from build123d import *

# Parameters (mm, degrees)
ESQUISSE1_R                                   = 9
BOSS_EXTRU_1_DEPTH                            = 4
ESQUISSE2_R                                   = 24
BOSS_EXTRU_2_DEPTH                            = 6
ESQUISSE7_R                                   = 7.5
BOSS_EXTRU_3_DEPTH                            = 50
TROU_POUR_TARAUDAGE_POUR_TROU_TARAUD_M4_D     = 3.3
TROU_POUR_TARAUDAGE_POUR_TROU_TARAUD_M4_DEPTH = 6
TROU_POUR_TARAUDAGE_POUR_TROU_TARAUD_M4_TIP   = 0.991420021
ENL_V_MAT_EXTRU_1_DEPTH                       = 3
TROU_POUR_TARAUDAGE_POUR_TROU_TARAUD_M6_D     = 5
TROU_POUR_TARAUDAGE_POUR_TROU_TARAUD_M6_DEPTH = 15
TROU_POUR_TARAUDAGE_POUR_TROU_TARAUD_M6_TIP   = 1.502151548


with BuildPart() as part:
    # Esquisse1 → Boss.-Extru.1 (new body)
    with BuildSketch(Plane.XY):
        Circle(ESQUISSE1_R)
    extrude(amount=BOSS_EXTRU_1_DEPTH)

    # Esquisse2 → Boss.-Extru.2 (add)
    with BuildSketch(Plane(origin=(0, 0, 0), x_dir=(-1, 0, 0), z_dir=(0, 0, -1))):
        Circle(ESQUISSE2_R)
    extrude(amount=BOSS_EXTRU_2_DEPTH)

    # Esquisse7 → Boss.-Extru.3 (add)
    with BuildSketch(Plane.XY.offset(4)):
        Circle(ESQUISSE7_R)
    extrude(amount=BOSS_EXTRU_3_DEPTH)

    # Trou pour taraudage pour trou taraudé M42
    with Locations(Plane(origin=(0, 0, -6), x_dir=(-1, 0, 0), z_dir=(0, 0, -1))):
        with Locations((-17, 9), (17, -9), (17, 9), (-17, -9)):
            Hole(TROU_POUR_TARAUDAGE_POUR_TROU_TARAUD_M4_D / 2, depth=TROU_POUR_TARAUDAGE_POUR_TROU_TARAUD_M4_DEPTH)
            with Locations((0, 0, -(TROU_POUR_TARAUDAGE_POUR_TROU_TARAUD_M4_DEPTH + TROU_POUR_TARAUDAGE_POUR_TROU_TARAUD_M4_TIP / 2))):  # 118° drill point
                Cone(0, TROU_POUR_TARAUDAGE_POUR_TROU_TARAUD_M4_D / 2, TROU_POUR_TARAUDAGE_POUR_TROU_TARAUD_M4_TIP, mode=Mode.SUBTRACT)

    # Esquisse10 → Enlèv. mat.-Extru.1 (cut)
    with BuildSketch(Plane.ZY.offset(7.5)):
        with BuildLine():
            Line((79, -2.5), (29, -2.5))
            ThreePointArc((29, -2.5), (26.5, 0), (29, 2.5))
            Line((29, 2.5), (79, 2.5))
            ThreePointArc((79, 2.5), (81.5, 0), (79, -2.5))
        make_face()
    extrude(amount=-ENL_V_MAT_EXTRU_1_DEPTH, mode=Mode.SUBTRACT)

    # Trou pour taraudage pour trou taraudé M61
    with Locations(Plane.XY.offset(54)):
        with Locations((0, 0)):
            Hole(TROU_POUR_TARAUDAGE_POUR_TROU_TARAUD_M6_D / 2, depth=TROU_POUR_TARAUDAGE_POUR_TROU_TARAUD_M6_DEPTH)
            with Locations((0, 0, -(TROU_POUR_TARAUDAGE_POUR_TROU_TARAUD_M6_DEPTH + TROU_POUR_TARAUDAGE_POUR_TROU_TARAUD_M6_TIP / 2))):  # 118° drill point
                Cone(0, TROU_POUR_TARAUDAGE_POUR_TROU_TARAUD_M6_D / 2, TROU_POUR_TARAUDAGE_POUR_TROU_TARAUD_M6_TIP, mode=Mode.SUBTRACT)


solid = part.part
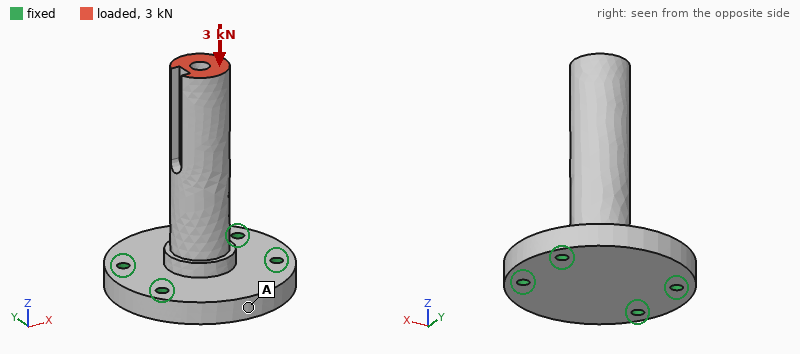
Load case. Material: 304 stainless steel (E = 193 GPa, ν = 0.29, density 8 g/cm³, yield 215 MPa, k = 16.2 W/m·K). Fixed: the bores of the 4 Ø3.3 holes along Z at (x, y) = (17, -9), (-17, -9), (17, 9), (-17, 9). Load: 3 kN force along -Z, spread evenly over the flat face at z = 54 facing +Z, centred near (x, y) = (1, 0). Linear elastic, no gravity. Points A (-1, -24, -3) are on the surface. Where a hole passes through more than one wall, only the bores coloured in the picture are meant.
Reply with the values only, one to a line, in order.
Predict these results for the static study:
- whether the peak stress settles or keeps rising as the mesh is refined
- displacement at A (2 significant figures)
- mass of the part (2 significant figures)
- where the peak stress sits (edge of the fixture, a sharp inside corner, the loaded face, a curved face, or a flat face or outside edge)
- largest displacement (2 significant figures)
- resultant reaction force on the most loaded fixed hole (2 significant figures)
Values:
keeps rising
2.4 µm
160 g
edge of the fixture
12 µm
810 N
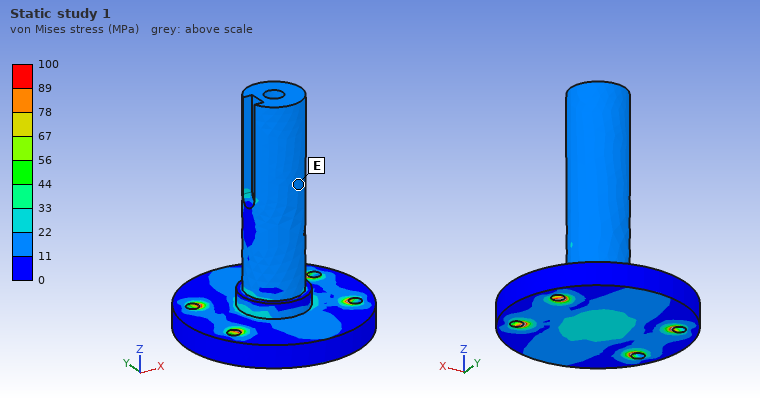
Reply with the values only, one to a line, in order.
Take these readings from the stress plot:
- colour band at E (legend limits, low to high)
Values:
11 to 22 MPa
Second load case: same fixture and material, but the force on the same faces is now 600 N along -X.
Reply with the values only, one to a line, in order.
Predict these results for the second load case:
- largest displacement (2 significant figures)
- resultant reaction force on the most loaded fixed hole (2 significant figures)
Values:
88 µm
650 N
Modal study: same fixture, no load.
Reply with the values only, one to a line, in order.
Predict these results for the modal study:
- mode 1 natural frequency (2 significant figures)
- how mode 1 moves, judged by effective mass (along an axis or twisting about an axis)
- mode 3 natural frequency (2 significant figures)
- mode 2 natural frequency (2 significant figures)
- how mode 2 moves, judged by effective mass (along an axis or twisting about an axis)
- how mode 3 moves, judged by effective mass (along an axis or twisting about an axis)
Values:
2900 Hz
along Y
12 kHz
3200 Hz
along X
along Z
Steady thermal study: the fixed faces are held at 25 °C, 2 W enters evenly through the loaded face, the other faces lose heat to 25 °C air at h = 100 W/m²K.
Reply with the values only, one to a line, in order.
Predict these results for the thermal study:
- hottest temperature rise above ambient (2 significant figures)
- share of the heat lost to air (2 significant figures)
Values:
16 K
90 %
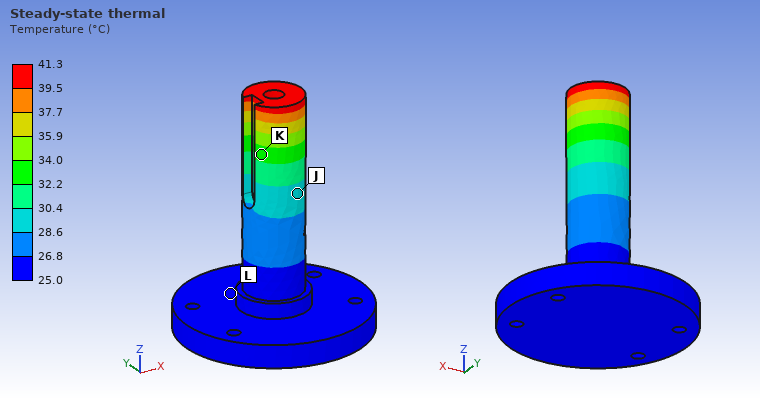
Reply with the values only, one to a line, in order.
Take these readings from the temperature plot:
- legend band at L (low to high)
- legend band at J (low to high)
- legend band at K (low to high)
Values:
25.0 to 26.8 °C
28.6 to 30.4 °C
32.2 to 34.0 °C
